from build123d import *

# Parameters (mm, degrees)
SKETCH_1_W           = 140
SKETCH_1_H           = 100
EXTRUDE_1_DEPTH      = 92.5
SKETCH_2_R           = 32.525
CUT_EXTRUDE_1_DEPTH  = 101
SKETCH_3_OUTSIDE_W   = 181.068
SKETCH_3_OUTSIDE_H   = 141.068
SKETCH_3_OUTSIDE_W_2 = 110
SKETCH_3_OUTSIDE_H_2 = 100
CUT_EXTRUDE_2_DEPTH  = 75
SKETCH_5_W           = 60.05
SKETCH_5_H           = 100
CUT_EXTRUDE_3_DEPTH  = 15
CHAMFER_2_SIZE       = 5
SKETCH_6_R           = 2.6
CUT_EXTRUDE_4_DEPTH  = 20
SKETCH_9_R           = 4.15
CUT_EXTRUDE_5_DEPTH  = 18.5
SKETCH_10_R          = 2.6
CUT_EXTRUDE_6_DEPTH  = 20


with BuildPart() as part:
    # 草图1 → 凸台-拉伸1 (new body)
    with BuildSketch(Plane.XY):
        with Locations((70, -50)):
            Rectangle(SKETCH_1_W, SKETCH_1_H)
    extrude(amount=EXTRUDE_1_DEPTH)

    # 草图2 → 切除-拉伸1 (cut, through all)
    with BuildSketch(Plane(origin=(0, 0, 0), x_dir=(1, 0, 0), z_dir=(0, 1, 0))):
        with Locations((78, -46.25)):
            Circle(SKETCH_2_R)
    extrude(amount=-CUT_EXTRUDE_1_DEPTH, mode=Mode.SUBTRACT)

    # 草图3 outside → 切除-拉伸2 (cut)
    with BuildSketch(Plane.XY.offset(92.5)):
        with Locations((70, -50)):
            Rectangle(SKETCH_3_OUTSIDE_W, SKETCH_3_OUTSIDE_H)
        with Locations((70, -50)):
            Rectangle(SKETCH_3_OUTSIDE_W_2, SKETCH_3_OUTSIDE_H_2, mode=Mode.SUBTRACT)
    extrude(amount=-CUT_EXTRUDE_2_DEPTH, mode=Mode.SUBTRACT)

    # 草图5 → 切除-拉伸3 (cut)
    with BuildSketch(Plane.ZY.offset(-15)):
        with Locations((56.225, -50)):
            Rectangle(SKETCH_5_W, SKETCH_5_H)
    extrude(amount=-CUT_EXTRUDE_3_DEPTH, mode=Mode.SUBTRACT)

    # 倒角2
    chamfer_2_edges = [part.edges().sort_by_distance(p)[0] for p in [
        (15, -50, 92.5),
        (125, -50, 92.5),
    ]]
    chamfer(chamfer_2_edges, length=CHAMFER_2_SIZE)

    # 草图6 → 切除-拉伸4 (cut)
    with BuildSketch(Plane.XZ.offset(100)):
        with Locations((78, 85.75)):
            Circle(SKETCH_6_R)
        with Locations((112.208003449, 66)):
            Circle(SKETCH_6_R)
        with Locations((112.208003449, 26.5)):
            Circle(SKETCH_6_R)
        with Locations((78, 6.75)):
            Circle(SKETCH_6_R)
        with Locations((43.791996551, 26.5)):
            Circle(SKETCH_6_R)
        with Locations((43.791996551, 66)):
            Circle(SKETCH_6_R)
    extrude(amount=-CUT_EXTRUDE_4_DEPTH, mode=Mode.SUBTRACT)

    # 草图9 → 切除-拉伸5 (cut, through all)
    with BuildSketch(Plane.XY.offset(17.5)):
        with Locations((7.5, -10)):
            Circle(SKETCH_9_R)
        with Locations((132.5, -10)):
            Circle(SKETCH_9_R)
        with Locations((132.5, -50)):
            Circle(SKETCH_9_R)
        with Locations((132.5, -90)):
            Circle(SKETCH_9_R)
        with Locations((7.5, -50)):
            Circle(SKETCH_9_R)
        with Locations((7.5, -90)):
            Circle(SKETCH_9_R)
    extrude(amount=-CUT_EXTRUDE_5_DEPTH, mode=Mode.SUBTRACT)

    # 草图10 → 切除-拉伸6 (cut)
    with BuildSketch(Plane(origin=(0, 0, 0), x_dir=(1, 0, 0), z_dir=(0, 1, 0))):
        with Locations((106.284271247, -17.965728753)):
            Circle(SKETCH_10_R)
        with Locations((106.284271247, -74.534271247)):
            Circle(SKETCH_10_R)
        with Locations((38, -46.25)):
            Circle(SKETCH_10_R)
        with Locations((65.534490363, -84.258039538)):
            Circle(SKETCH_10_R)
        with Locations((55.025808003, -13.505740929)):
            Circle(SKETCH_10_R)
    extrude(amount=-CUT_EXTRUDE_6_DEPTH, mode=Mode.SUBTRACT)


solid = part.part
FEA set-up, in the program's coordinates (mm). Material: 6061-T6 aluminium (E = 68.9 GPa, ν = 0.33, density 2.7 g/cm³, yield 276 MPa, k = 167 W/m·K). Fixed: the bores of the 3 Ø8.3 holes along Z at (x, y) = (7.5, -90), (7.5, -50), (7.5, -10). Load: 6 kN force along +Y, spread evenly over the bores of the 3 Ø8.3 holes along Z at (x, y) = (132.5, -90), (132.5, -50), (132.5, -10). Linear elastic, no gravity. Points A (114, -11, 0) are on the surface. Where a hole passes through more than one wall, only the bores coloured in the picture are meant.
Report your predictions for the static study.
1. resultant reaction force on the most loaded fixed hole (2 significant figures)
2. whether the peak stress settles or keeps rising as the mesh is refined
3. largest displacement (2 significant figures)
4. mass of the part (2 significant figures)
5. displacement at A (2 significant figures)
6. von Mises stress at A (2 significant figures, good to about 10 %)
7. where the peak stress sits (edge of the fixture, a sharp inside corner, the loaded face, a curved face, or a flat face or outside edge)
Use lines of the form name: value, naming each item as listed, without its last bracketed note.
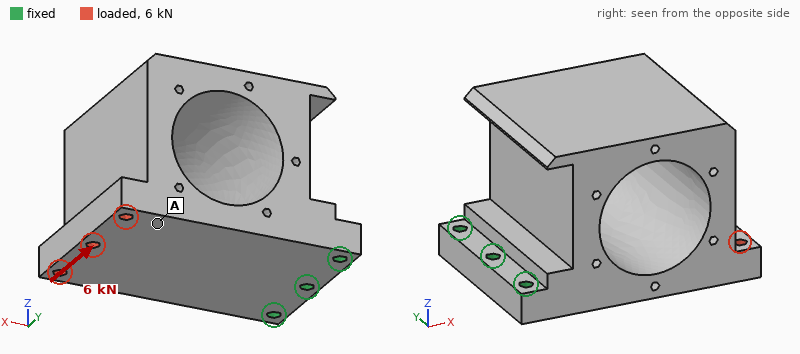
resultant reaction force on the most loaded fixed hole: 9.3 kN
whether the peak stress settles or keeps rising as the mesh is refined: keeps rising
largest displacement: 69 µm
mass of the part: 1.7 kg
displacement at A: 50 µm
von Mises stress at A: 5.3 MPa
where the peak stress sits: edge of the fixture
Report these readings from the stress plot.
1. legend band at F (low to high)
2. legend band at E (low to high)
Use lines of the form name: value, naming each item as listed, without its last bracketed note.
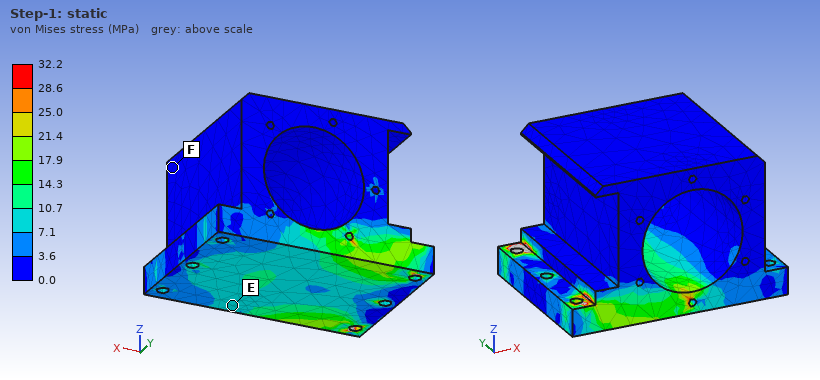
legend band at F: 0.0 to 3.6 MPa
legend band at E: 7.1 to 10.7 MPa
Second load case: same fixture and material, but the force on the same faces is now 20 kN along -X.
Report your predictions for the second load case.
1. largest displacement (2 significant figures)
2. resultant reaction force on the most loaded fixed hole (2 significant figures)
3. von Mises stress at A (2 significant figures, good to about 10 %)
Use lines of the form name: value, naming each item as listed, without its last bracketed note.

largest displacement: 40 µm
resultant reaction force on the most loaded fixed hole: 7.2 kN
von Mises stress at A: 17 MPa
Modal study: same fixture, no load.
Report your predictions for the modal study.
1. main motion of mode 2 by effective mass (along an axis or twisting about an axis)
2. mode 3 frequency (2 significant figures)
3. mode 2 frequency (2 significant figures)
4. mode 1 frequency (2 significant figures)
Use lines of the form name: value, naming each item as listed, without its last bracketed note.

main motion of mode 2 by effective mass: along Y
mode 3 frequency: 2600 Hz
mode 2 frequency: 1700 Hz
mode 1 frequency: 530 Hz
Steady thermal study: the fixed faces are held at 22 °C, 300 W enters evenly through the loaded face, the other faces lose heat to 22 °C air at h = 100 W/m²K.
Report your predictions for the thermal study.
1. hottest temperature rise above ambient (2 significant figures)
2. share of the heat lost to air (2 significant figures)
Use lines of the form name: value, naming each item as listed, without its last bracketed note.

hottest temperature rise above ambient: 69 K
share of the heat lost to air: 62 %
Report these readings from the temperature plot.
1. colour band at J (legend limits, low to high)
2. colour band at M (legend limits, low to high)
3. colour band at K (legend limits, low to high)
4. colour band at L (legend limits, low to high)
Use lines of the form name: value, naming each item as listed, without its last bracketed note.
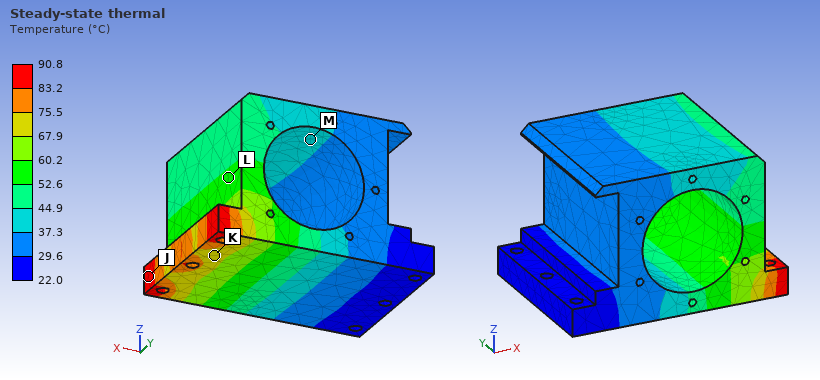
colour band at J: 83.2 to 90.8 °C
colour band at M: 37.3 to 44.9 °C
colour band at K: 67.9 to 75.5 °C
colour band at L: 52.6 to 60.2 °C
